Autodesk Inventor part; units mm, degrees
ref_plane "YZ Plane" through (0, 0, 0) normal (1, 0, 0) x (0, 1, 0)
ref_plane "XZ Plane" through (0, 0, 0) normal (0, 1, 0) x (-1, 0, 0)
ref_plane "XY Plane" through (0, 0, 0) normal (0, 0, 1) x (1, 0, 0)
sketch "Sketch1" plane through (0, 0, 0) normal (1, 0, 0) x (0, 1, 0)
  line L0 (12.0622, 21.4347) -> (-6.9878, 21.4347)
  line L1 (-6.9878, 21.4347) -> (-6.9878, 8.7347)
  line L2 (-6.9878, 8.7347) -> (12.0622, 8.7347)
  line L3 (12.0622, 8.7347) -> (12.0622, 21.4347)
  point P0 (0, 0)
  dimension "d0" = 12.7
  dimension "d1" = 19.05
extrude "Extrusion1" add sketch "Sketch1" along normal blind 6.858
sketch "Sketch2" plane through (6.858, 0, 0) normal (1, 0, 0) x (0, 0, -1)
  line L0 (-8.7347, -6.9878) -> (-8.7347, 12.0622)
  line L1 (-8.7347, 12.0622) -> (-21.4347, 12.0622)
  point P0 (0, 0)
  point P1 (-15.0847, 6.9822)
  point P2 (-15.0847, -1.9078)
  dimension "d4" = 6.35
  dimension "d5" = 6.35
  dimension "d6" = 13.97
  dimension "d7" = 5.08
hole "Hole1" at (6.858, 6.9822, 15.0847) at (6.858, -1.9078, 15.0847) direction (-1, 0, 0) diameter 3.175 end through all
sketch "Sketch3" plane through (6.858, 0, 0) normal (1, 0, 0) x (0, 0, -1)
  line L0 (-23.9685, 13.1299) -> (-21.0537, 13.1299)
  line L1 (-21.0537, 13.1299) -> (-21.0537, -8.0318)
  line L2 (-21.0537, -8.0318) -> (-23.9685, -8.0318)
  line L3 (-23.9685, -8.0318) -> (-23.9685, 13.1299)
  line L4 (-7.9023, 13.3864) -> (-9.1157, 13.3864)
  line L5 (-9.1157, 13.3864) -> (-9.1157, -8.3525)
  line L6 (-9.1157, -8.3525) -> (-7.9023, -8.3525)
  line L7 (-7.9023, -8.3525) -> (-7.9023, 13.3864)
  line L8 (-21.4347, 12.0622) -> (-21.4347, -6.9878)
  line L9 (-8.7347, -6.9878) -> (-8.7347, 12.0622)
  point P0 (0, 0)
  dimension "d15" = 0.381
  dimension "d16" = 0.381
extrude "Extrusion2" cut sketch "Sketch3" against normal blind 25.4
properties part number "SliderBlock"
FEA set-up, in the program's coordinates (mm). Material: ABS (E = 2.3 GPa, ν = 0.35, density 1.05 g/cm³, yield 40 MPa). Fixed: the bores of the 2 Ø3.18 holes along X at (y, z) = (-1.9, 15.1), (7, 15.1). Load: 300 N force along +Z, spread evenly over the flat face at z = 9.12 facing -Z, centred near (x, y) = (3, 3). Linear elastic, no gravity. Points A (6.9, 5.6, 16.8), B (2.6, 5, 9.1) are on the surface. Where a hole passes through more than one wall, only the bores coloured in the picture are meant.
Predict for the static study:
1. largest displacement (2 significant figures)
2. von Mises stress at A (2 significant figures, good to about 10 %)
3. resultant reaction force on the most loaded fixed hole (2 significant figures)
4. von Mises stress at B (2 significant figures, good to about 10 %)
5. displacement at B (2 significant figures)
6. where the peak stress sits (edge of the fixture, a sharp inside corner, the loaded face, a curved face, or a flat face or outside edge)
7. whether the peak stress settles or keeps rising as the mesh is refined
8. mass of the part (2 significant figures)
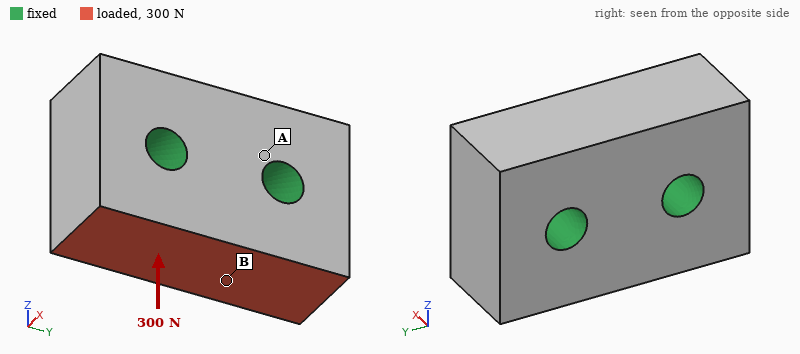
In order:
11 µm
0.78 MPa
150 N
2.7 MPa
5.4 µm
edge of the fixture
keeps rising
1.5 g
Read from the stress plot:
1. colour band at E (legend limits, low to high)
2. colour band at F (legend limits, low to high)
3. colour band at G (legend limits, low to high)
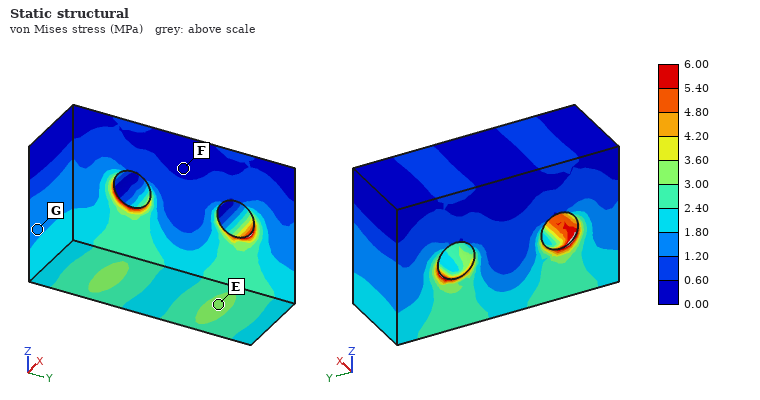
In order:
3.00 to 3.60 MPa
0.00 to 0.60 MPa
1.20 to 1.80 MPa
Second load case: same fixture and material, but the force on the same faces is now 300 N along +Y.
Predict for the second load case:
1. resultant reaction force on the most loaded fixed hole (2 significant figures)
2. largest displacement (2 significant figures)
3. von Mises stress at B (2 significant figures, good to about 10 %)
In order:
200 N
36 µm
4.6 MPa
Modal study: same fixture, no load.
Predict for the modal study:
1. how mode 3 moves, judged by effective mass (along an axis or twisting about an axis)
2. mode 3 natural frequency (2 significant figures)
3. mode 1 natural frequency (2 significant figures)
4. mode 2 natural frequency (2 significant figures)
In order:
twisting about Z
30 kHz
27 kHz
28 kHz
